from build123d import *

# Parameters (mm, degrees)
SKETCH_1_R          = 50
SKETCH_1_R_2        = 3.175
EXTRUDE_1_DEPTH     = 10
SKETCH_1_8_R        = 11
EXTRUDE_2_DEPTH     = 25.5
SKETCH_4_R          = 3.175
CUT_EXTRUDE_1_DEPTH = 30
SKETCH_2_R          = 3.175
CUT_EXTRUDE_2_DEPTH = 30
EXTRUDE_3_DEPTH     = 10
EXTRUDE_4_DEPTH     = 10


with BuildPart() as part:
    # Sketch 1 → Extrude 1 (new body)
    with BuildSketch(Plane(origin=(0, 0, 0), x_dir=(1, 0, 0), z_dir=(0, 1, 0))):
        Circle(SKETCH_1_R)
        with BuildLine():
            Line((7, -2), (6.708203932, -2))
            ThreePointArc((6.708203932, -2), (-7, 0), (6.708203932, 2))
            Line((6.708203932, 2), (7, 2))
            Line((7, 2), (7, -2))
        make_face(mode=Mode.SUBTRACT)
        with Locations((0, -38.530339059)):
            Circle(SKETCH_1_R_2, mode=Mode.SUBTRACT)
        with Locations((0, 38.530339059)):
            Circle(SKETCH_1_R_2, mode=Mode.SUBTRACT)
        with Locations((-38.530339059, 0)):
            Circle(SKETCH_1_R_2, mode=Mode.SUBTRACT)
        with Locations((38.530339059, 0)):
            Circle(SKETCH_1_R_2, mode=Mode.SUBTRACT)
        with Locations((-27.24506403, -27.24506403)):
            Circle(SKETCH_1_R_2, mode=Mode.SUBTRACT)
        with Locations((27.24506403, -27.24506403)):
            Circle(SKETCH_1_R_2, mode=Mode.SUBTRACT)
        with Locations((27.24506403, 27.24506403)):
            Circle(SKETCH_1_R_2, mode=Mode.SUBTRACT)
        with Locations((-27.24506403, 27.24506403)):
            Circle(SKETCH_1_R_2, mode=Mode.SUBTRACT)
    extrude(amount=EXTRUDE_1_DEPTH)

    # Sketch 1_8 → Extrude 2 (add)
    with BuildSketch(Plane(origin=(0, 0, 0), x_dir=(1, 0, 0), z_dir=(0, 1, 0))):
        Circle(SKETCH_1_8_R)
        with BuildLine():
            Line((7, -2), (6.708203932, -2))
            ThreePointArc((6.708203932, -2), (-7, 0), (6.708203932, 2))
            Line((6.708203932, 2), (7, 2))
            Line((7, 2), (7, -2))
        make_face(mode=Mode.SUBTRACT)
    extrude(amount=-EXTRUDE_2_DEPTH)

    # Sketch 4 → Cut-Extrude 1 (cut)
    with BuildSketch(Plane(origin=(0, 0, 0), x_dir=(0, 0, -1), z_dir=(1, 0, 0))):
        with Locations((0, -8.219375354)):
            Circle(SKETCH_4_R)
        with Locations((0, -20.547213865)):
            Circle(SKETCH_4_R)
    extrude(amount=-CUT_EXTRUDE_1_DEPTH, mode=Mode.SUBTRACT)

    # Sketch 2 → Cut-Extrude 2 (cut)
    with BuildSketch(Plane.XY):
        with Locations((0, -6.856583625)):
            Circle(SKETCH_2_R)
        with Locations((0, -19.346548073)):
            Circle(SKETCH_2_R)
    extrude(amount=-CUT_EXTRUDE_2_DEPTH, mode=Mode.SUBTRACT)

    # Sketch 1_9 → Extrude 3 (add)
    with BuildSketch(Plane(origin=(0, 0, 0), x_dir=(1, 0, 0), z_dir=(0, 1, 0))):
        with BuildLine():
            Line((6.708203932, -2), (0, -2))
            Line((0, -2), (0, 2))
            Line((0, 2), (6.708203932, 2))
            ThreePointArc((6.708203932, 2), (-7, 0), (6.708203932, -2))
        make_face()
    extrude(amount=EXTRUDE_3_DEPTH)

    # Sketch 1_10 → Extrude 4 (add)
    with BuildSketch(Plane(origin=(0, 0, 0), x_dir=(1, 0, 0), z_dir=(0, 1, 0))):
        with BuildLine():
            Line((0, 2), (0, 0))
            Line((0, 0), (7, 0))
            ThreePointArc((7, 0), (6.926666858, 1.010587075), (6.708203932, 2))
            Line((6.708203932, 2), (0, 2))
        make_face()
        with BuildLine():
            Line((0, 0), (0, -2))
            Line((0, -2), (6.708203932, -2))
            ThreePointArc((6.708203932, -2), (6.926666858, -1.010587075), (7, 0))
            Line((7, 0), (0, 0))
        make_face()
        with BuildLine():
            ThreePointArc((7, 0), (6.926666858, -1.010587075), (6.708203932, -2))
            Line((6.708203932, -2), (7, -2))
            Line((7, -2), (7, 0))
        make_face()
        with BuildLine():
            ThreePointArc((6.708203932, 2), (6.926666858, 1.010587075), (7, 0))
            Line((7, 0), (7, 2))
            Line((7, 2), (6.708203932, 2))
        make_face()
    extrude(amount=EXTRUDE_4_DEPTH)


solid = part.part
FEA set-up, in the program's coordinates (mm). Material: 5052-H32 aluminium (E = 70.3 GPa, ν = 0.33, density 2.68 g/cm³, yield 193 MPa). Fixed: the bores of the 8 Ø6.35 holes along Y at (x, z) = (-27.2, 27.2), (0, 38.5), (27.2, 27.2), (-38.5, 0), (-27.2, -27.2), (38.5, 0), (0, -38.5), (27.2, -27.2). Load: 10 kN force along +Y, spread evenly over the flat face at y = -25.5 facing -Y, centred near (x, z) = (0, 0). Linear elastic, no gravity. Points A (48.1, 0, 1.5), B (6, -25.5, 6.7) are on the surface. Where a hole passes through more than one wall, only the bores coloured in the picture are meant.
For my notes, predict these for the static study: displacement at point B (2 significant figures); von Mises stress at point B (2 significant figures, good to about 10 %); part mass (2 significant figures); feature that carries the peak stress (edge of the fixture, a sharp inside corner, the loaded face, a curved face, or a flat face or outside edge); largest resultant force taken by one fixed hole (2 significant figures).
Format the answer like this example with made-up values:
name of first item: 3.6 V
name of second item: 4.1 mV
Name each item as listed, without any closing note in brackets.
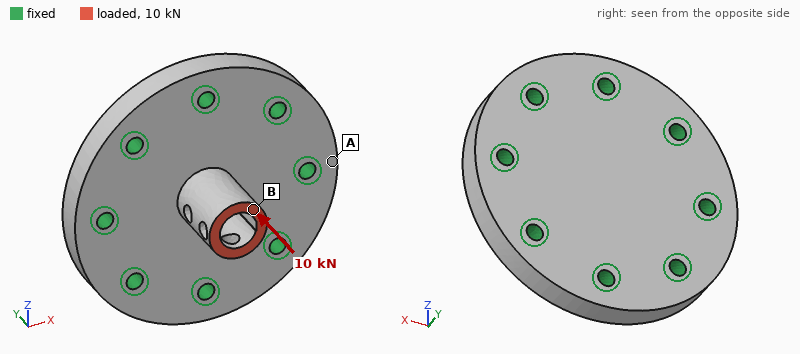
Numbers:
displacement at point B: 52 µm
von Mises stress at point B: 43 MPa
part mass: 220 g
feature that carries the peak stress: a curved face
largest resultant force taken by one fixed hole: 1.3 kN
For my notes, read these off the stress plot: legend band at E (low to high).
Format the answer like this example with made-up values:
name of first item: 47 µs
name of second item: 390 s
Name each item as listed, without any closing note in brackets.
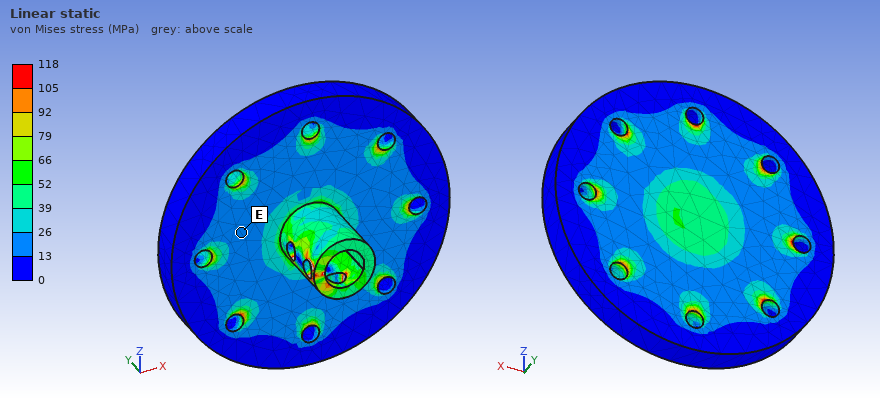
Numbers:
legend band at E: 13 to 26 MPa
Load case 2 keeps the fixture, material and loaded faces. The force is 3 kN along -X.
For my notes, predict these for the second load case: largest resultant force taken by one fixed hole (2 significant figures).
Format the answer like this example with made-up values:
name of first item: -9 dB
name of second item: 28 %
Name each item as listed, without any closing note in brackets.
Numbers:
largest resultant force taken by one fixed hole: 1.0 kN
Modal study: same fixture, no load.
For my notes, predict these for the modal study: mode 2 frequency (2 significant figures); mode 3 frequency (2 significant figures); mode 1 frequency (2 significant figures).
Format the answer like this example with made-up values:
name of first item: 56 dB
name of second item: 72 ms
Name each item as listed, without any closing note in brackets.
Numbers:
mode 2 frequency: 12 kHz
mode 3 frequency: 12 kHz
mode 1 frequency: 12 kHz
